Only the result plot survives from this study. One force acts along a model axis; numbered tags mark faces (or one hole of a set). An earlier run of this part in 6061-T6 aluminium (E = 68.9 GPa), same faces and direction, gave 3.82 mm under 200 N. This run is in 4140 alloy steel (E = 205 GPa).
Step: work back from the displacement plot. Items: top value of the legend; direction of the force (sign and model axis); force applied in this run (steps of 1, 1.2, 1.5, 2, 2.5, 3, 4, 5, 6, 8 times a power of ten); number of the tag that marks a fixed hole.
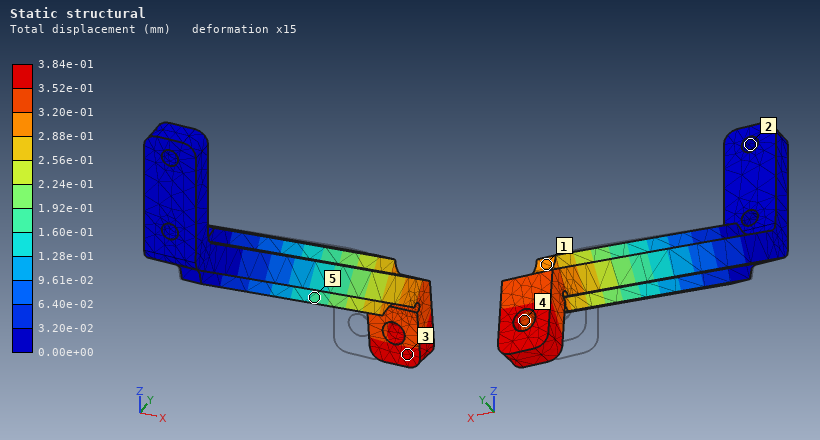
3.84e-01 mm
+X
60 N
2
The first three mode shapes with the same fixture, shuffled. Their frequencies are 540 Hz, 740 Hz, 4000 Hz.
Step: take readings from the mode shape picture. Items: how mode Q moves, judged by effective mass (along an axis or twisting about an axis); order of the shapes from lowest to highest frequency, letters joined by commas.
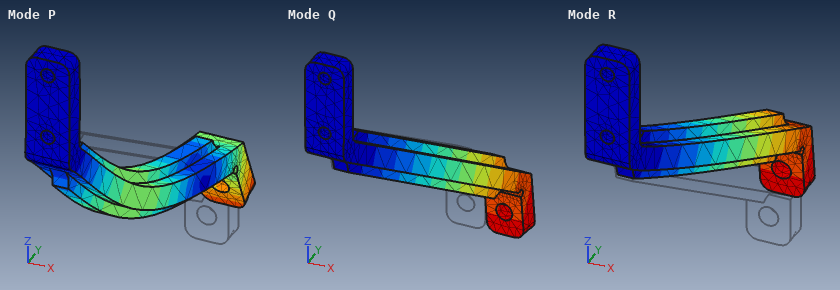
along X
R, Q, P
